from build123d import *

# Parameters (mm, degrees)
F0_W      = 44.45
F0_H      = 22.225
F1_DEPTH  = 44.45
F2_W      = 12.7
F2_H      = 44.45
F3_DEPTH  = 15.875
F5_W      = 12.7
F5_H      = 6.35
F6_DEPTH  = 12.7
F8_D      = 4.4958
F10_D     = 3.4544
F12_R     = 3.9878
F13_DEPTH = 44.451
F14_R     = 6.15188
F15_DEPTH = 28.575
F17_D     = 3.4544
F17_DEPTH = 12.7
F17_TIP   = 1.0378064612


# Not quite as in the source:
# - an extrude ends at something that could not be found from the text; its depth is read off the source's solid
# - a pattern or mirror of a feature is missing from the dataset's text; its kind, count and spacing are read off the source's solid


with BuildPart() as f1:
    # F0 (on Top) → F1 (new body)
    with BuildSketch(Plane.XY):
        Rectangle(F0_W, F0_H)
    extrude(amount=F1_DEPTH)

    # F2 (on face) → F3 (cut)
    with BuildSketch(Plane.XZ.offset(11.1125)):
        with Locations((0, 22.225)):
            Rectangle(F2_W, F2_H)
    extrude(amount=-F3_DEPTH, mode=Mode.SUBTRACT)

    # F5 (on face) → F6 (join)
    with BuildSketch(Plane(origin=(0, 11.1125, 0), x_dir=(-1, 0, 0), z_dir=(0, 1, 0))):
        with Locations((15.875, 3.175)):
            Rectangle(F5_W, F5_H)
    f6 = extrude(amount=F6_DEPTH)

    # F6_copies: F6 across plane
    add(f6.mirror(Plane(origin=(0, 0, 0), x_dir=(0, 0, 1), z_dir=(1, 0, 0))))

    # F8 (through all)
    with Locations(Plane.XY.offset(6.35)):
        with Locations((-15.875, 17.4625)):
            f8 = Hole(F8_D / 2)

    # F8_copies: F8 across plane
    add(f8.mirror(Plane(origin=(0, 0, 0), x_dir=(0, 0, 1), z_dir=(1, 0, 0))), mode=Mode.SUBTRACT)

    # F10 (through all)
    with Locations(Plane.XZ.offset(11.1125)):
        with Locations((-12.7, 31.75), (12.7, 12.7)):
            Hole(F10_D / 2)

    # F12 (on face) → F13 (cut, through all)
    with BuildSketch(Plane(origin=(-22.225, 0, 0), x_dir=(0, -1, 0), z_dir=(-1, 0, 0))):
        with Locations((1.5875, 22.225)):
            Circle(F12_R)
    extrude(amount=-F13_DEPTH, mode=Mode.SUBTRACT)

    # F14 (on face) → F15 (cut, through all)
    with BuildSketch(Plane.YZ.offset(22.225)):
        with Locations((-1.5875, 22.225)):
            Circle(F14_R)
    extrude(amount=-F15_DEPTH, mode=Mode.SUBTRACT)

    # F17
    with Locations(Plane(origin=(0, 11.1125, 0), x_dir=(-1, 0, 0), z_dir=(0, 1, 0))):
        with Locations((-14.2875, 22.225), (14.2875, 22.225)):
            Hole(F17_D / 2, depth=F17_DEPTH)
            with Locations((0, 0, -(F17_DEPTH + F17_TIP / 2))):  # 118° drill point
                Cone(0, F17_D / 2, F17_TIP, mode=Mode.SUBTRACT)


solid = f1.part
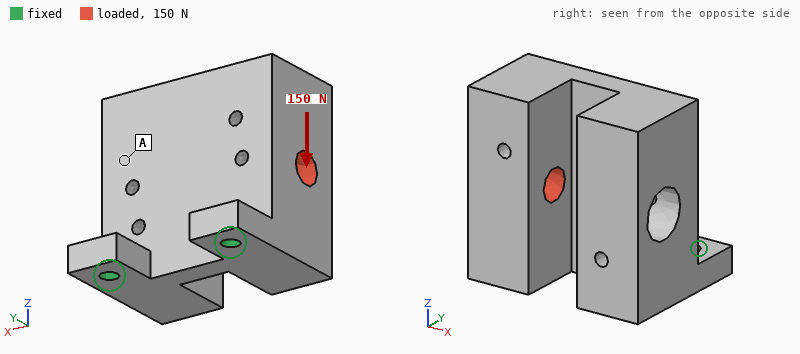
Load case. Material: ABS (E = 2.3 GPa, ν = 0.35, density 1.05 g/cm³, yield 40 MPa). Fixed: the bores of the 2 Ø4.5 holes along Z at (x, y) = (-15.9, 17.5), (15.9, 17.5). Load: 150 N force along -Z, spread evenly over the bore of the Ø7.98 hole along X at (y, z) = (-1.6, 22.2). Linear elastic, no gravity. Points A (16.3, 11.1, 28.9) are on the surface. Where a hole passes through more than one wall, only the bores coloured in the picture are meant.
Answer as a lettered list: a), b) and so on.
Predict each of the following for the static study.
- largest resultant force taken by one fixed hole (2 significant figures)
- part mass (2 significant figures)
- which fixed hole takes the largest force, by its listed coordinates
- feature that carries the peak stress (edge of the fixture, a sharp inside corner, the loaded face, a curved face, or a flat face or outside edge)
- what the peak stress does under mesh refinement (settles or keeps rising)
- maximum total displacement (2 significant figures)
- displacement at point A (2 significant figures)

a) 140 N
b) 35 g
c) (-15.9, 17.5)
d) edge of the fixture
e) keeps rising
f) 0.77 mm
g) 0.35 mm
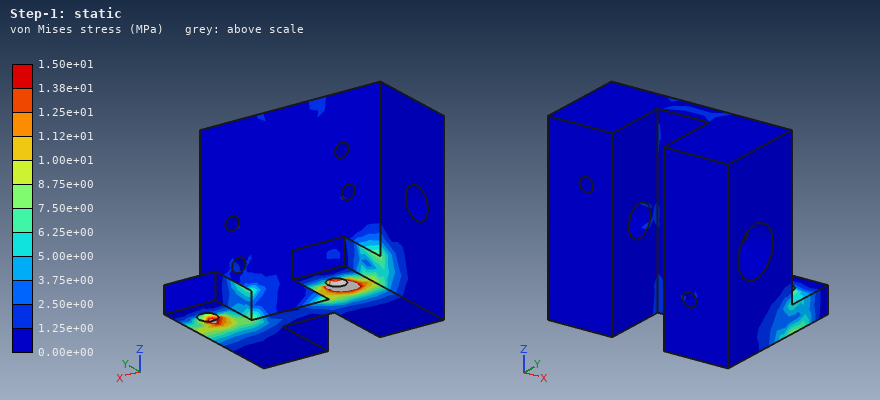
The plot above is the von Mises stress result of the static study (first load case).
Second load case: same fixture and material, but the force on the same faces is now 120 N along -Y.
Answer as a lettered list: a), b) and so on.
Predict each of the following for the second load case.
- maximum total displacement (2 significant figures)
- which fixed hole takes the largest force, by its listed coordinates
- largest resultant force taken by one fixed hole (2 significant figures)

a) 0.80 mm
b) (-15.9, 17.5)
c) 110 N
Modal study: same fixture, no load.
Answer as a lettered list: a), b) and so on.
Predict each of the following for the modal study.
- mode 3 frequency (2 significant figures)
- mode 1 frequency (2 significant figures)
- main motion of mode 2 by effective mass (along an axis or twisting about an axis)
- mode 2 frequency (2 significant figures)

a) 1400 Hz
b) 390 Hz
c) along X
d) 1300 Hz
